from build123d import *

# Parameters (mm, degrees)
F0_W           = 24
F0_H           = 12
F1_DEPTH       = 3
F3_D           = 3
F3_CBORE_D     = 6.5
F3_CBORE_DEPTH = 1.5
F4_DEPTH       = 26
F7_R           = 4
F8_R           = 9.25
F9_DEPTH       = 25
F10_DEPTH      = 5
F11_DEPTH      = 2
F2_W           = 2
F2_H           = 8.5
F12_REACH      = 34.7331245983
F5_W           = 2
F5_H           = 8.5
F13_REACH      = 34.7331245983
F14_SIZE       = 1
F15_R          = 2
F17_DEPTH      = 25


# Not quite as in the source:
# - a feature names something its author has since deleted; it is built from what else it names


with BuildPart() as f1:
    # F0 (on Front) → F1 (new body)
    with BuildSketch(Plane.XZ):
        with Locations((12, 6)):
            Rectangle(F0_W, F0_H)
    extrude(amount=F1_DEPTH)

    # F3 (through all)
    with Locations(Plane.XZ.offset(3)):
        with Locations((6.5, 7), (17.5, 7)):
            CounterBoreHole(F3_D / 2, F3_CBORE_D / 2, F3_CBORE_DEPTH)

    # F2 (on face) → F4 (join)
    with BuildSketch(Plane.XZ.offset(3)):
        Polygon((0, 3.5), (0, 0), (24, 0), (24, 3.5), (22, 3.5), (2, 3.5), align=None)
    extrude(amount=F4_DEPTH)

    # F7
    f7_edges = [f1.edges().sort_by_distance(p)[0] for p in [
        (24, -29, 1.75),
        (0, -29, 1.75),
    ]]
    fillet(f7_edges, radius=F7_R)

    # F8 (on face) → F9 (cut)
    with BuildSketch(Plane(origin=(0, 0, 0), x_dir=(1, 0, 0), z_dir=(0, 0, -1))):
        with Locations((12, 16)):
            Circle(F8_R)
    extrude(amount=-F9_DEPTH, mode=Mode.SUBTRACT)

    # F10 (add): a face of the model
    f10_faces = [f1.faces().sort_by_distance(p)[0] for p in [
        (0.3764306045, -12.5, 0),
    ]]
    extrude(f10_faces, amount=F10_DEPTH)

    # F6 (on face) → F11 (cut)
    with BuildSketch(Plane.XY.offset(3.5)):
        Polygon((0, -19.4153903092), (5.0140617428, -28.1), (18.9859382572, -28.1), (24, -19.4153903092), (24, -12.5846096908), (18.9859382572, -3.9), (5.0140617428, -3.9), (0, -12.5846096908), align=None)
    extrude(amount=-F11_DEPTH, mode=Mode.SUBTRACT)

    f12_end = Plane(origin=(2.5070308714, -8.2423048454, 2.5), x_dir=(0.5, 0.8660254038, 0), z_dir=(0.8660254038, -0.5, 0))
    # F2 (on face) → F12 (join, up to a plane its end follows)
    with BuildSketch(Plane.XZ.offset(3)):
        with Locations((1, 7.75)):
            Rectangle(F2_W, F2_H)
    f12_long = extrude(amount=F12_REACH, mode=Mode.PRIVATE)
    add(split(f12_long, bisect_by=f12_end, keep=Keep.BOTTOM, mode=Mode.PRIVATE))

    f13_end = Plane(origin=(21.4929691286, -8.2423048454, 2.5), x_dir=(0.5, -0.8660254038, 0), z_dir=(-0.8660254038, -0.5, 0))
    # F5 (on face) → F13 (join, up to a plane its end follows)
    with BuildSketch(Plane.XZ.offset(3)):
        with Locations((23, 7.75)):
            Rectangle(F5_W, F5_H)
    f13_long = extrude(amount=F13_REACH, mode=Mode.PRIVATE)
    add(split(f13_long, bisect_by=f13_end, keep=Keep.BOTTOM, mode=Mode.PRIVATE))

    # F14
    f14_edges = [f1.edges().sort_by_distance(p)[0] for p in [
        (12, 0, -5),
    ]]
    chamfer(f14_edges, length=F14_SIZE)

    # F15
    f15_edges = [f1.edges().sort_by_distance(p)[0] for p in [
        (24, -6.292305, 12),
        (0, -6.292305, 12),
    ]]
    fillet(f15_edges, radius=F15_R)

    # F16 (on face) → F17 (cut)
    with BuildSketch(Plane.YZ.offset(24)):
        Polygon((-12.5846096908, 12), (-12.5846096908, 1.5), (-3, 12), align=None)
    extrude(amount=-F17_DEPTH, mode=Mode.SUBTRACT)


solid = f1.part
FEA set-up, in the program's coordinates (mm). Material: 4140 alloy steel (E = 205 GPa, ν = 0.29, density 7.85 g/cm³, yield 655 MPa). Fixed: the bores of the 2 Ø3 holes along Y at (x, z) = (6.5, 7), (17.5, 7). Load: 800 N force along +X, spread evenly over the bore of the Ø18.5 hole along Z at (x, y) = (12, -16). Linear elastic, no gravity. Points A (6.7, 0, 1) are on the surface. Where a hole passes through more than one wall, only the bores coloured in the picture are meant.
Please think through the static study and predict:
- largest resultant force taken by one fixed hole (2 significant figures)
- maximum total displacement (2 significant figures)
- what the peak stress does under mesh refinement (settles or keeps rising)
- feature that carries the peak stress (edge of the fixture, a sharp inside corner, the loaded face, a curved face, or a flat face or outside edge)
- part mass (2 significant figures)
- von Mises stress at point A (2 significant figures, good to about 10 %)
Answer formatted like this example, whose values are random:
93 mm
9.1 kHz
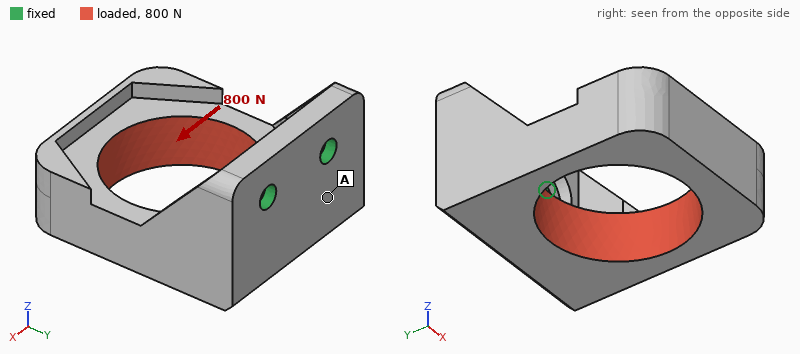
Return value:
1.1 kN
68 µm
keeps rising
edge of the fixture
29 g
52 MPa
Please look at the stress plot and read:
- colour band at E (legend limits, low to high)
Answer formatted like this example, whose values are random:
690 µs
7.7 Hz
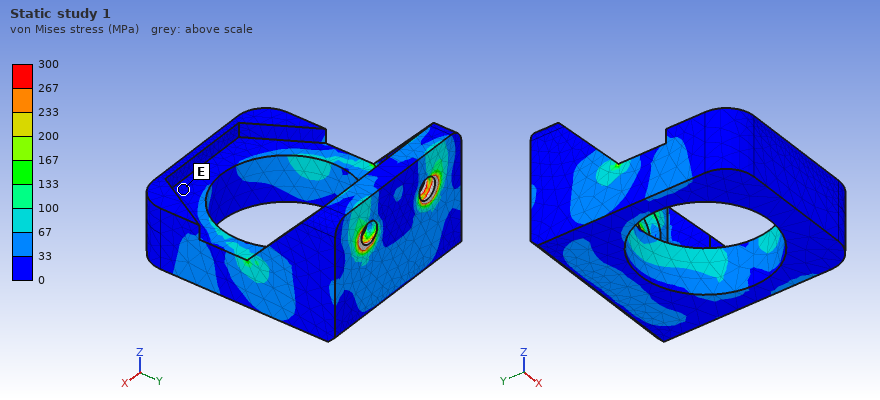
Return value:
0 to 33 MPa
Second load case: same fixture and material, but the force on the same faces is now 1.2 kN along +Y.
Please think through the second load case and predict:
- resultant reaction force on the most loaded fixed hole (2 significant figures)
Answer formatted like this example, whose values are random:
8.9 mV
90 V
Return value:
600 N
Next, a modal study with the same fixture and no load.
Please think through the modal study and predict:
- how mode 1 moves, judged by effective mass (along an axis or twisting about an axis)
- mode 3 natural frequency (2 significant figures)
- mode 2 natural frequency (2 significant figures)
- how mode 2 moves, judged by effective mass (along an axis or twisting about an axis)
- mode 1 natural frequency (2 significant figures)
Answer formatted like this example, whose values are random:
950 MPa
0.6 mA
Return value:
along Z
9800 Hz
4300 Hz
along X
2200 Hz
